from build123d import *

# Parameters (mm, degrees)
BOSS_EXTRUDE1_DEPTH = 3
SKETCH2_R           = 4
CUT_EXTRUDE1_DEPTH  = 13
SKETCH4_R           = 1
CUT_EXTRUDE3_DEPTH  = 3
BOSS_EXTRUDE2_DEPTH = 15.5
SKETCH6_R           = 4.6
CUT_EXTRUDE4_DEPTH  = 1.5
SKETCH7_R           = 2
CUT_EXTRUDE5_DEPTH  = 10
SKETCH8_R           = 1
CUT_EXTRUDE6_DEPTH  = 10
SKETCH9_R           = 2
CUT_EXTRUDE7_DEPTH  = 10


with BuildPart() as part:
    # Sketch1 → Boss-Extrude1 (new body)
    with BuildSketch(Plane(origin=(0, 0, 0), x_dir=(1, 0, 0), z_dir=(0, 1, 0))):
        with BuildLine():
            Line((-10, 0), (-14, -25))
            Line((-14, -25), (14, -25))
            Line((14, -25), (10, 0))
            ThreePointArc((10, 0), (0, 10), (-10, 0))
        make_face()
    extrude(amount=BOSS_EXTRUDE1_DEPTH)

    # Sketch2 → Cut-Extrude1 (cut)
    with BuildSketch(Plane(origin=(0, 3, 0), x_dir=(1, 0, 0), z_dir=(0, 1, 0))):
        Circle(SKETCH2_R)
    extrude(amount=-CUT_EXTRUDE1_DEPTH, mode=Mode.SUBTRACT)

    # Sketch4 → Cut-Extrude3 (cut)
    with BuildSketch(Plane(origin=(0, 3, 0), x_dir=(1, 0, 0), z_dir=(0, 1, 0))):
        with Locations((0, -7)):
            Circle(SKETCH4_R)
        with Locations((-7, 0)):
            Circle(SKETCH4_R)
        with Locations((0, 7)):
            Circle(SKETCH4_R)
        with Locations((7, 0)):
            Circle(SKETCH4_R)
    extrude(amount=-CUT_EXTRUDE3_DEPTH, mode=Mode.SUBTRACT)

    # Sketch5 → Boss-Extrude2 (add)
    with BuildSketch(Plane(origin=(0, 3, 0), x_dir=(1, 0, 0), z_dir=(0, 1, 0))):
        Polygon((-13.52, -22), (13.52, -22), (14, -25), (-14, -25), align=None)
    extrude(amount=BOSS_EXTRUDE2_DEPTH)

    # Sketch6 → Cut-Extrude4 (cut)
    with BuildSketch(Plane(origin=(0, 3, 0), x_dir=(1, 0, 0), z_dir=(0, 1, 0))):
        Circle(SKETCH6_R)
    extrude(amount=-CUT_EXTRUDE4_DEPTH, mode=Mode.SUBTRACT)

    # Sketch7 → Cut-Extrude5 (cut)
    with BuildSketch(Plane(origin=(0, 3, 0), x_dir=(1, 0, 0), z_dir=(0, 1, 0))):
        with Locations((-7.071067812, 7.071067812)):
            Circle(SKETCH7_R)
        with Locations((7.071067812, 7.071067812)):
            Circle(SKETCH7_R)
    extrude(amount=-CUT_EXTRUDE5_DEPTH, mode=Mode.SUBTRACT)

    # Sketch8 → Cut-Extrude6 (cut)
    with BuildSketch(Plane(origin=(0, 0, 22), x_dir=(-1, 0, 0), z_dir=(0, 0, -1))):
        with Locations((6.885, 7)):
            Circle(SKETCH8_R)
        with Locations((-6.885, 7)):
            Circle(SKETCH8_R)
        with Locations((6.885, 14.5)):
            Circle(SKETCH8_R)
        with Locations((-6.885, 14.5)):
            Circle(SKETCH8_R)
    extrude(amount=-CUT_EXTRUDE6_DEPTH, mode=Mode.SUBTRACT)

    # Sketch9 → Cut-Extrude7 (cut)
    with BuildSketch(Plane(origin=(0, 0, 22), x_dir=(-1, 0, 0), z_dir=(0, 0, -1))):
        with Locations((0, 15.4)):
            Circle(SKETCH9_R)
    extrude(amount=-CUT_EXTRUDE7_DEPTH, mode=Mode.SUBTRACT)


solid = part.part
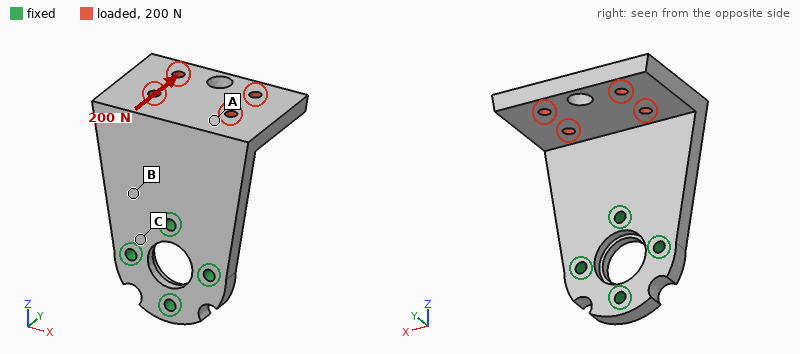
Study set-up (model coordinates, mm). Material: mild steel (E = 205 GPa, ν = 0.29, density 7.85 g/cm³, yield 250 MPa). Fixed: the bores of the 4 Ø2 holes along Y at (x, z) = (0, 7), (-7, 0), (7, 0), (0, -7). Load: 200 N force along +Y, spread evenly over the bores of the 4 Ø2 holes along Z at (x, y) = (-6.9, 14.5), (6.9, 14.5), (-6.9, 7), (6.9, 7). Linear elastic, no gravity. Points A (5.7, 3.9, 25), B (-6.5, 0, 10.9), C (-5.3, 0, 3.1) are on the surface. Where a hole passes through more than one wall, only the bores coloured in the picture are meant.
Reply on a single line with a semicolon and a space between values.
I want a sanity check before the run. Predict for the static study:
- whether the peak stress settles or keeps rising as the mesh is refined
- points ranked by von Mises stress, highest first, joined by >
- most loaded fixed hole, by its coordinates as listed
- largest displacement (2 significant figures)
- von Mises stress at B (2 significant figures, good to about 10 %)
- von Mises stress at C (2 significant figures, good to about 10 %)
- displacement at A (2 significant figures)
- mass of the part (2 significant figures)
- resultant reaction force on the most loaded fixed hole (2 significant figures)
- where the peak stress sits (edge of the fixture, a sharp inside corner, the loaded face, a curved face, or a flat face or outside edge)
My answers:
keeps rising; B > C > A; (0, 7); 62 µm; 61 MPa; 29 MPa; 40 µm; 25 g; 390 N; edge of the fixture
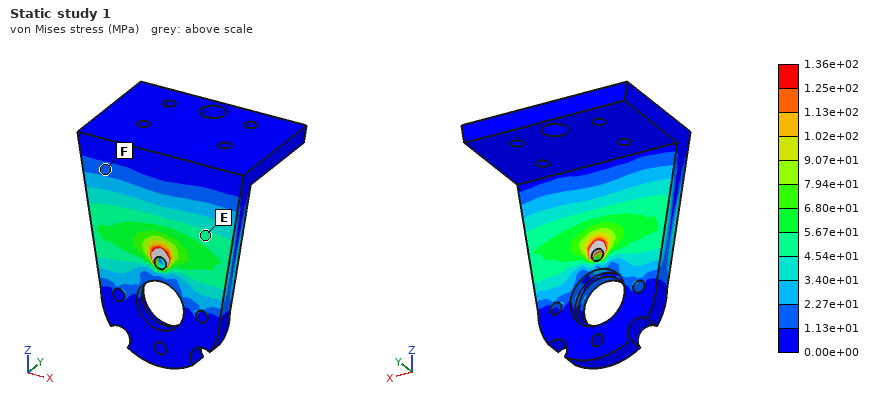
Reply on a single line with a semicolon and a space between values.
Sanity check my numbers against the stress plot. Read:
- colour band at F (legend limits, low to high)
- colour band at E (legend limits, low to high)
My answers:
1.13e+01 to 2.27e+01 MPa; 4.54e+01 to 5.67e+01 MPa
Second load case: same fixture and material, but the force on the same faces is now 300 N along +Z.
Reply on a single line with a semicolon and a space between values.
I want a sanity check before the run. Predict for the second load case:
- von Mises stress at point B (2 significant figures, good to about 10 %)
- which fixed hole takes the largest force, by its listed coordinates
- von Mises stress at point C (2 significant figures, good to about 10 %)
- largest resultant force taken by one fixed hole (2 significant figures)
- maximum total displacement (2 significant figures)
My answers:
66 MPa; (0, 7); 17 MPa; 270 N; 95 µm
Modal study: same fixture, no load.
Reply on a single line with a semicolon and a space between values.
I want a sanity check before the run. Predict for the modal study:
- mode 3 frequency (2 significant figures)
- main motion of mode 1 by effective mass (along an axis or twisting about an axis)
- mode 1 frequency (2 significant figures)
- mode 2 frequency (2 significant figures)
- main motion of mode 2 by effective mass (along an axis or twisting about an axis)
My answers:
7500 Hz; along Y; 2600 Hz; 3800 Hz; along X
